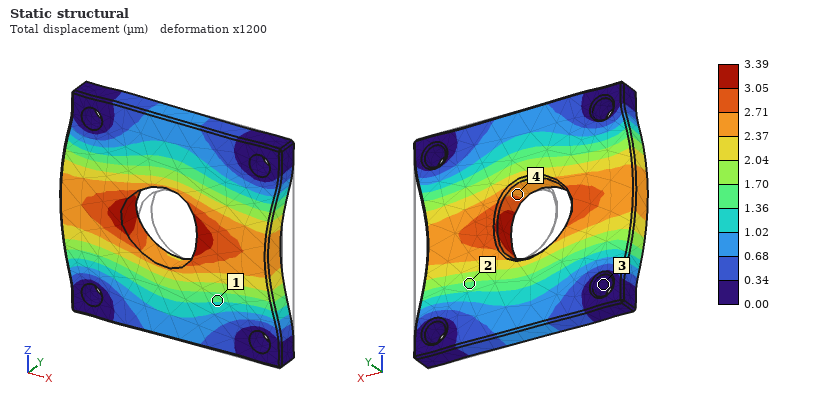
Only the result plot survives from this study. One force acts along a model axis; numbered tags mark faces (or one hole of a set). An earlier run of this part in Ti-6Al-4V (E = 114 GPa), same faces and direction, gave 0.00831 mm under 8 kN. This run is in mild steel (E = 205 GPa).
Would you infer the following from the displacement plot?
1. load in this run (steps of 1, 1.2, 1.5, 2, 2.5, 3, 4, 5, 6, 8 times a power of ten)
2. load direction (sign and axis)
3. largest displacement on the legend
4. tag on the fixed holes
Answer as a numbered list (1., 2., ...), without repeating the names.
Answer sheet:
1. 6 kN
2. -X
3. 3.39 µm
4. 3
